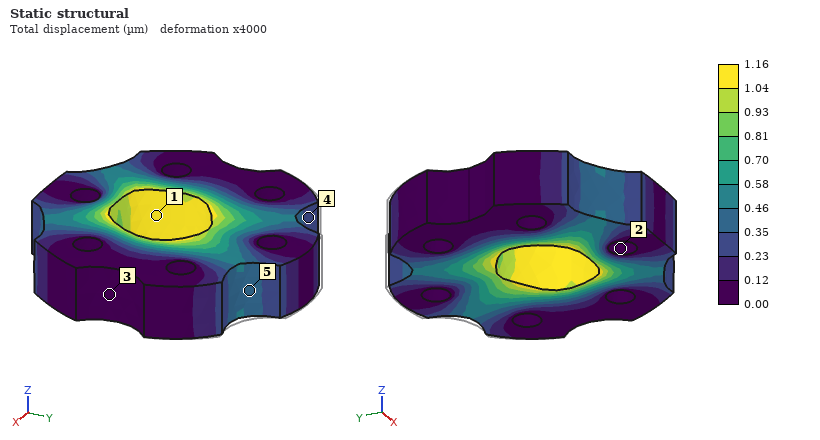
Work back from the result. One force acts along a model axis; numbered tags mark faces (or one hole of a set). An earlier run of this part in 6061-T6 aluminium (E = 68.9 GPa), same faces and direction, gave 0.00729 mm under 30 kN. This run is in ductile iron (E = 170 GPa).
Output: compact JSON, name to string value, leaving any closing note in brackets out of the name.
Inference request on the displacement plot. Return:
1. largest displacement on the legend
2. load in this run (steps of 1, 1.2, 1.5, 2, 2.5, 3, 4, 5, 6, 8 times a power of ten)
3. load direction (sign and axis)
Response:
{"largest displacement on the legend": "1.16 µm", "load in this run": "12 kN", "load direction": "-Y"}
